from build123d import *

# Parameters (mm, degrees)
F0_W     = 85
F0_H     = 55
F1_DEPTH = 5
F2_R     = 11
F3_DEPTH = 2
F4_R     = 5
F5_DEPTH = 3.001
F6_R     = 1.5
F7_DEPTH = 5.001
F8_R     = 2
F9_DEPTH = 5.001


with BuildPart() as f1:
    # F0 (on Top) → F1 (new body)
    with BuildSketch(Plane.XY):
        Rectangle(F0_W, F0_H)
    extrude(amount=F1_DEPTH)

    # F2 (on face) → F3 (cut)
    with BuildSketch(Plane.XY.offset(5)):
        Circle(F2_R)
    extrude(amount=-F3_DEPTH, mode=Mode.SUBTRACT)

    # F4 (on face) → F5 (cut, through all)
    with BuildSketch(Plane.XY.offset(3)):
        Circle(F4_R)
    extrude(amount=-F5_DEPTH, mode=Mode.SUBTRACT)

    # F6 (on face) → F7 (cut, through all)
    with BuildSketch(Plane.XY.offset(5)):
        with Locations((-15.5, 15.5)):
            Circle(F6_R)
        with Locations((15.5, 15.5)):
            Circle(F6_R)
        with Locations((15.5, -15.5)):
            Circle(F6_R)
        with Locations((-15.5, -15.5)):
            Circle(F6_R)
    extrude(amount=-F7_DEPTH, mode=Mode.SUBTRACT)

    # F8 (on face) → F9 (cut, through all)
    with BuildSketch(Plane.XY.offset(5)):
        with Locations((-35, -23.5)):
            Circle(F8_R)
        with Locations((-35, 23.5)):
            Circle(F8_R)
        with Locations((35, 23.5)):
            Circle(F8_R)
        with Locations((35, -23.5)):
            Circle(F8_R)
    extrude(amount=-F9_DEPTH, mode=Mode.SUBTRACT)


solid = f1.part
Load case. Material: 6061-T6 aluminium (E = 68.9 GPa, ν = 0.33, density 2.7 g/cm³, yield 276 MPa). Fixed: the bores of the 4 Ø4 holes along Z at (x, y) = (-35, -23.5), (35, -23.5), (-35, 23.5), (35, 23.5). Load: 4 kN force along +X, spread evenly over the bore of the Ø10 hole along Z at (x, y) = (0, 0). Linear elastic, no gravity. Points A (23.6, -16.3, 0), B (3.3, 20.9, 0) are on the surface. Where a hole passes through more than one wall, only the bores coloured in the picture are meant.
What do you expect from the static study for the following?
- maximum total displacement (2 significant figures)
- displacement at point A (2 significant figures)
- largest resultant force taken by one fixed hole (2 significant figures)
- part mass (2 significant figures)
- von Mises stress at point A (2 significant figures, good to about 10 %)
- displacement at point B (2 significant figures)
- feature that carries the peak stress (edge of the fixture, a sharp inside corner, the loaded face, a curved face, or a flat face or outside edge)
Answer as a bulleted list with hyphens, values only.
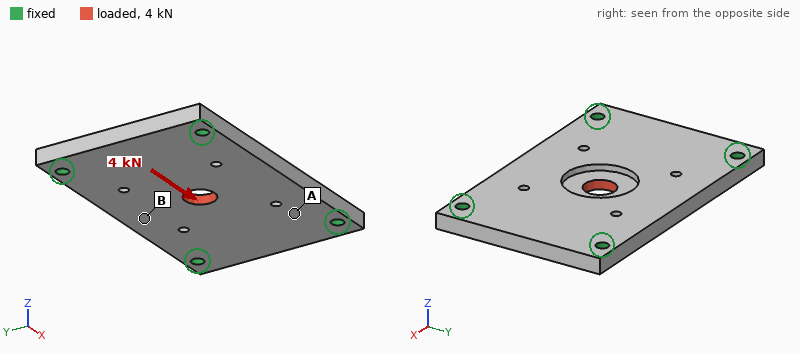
- 12 µm
- 3.3 µm
- 1.1 kN
- 59 g
- 14 MPa
- 4.2 µm
- the loaded face
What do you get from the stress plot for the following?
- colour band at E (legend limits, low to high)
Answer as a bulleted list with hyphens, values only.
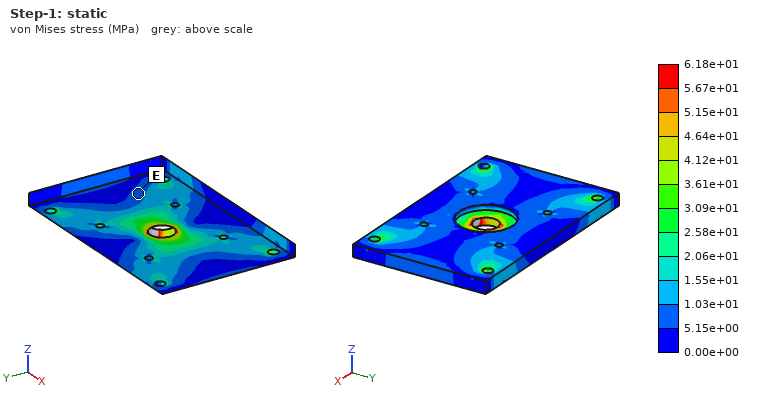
- 5.15e+00 to 1.03e+01 MPa
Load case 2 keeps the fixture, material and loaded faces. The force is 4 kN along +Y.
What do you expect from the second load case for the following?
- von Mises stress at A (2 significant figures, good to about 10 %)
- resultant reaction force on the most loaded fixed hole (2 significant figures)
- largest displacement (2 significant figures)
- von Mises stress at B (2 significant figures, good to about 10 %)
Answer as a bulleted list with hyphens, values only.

- 20 MPa
- 1.3 kN
- 18 µm
- 8.5 MPa
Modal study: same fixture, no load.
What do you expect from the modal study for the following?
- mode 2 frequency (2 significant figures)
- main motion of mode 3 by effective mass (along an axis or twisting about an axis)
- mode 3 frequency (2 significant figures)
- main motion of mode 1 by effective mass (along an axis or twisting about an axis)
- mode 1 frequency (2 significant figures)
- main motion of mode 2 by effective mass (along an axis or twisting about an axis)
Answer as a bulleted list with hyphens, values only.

- 6600 Hz
- twisting about Y
- 9700 Hz
- along Z
- 4300 Hz
- twisting about X
